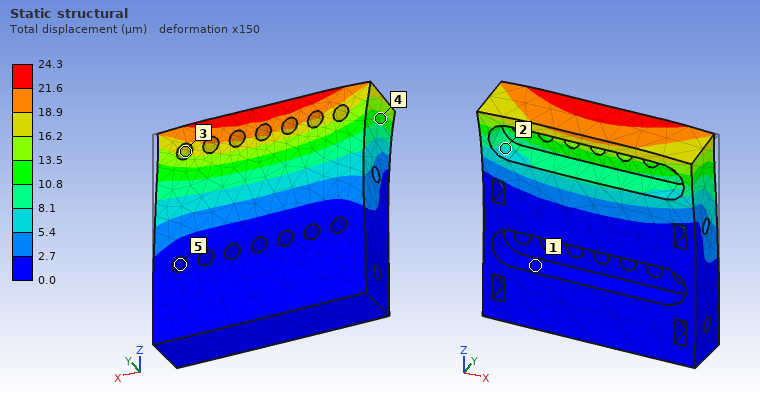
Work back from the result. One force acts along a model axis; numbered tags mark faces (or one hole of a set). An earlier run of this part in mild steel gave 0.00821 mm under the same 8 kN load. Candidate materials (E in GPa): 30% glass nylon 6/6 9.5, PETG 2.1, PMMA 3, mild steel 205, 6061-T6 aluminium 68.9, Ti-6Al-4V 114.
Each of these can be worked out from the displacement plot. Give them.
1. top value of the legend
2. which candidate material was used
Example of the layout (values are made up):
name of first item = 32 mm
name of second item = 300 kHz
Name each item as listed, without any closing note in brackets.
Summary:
top value of the legend = 24.3 µm
which candidate material was used = 6061-T6 aluminium
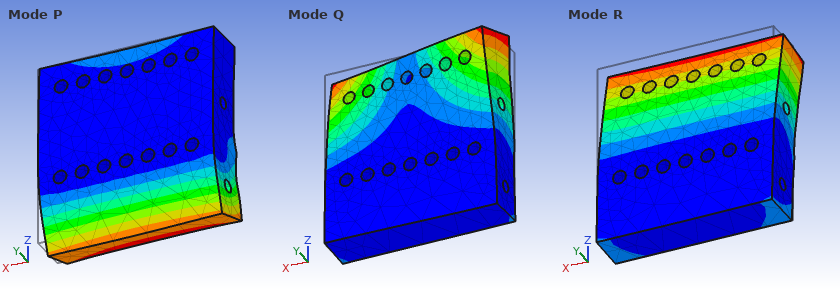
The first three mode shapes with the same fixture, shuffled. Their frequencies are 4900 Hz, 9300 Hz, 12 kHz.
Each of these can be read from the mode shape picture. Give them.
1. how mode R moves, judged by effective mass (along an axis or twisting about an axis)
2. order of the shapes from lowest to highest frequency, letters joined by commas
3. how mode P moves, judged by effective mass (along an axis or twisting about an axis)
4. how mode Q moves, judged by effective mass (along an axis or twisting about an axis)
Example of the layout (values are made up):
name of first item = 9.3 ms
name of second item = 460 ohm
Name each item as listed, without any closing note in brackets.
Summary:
how mode R moves, judged by effective mass = along Y
order of the shapes from lowest to highest frequency, letters joined by commas = R, Q, P
how mode P moves, judged by effective mass = along Y
how mode Q moves, judged by effective mass = twisting about Z
